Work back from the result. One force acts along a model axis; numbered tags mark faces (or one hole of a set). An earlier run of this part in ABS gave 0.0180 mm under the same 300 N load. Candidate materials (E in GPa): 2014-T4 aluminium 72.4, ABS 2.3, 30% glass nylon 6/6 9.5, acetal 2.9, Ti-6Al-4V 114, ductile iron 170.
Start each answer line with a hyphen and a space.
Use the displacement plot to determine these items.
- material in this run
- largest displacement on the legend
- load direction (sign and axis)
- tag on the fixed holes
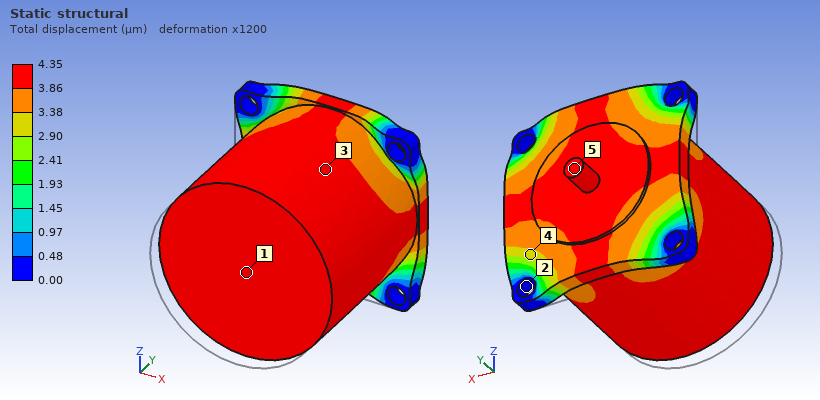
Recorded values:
- 30% glass nylon 6/6
- 4.35 µm
- +Y
- 2
